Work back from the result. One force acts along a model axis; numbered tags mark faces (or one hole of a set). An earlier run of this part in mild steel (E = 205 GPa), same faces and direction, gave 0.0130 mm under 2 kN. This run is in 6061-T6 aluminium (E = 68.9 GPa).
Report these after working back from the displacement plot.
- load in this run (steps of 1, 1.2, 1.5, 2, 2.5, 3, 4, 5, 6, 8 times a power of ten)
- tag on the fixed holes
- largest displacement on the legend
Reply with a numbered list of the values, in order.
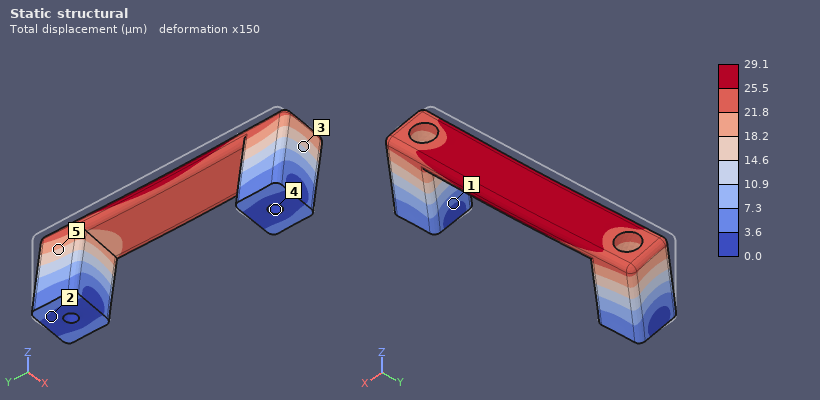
1. 1.5 kN
2. 4
3. 29.1 µm
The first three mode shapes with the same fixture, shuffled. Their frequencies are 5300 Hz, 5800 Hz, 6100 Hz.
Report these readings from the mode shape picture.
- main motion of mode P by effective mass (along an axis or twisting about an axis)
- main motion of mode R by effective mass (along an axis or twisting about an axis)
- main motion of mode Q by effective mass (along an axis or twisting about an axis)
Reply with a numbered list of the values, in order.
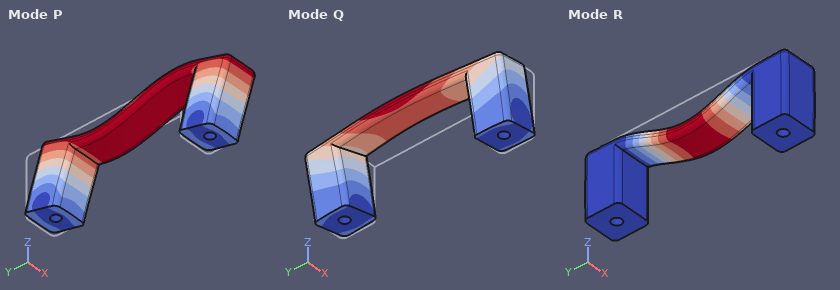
1. along Y
2. along Z
3. along X
